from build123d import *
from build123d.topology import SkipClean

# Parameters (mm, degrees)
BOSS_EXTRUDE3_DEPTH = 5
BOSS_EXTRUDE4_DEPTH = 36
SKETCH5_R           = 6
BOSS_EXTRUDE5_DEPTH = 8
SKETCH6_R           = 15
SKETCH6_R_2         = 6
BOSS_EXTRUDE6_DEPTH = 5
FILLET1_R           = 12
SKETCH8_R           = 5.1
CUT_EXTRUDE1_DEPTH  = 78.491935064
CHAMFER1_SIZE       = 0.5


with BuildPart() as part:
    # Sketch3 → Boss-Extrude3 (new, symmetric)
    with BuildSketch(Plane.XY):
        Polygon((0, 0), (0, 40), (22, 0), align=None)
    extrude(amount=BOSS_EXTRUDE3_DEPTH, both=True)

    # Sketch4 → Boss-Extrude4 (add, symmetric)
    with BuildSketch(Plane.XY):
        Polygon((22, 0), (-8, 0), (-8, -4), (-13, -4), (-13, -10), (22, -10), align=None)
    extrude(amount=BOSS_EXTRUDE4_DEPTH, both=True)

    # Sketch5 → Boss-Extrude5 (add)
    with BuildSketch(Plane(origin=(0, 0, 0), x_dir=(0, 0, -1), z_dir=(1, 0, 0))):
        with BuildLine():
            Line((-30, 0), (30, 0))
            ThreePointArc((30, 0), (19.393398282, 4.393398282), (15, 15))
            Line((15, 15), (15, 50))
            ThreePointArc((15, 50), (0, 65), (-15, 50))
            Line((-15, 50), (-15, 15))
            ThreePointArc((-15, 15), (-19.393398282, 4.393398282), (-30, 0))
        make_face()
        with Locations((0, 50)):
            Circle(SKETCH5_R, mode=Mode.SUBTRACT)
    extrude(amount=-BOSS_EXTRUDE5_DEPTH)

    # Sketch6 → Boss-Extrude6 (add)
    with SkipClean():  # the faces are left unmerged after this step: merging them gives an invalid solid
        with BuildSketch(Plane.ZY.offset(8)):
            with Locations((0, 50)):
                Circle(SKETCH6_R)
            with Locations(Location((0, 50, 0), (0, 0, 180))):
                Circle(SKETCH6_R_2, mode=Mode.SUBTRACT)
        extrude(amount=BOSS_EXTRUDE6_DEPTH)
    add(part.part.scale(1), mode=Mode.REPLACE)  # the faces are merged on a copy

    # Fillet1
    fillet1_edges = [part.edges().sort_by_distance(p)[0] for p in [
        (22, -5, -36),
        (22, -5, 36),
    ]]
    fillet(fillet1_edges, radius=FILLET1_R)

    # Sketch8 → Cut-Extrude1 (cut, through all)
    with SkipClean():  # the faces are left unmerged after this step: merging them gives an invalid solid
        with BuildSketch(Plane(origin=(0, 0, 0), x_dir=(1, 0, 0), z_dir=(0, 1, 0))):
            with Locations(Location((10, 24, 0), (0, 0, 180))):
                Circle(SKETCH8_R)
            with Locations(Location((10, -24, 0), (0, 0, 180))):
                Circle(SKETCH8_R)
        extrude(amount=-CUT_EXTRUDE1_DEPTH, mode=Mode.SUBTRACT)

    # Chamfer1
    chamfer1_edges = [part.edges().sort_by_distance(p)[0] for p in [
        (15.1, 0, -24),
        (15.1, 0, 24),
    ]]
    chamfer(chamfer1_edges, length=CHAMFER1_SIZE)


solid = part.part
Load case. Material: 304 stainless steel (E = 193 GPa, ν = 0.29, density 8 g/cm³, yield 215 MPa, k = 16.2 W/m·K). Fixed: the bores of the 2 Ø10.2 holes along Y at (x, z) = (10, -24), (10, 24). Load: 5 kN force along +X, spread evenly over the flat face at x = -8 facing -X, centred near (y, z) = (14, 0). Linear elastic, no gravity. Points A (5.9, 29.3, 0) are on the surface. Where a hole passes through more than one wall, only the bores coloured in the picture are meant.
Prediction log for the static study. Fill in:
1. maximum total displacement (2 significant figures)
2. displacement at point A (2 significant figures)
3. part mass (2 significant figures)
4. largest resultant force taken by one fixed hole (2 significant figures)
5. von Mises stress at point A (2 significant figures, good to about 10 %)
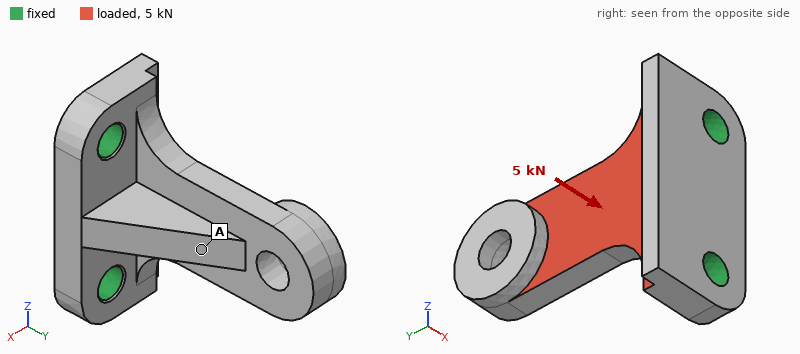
82 µm
38 µm
350 g
2.5 kN
18 MPa
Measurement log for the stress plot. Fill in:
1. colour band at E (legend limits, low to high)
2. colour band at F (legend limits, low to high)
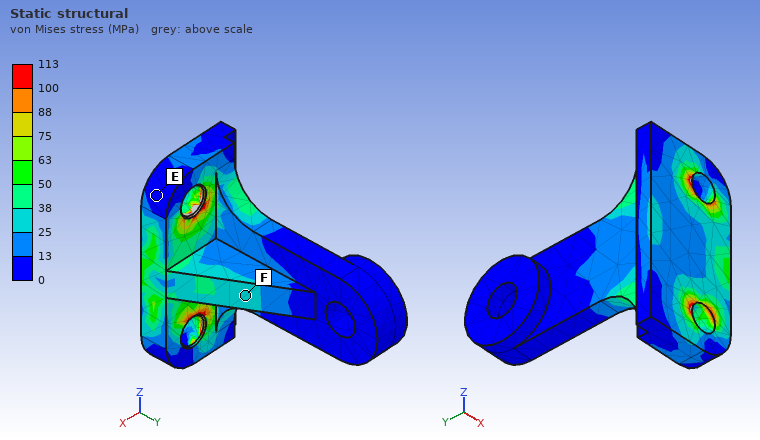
0 to 13 MPa
25 to 38 MPa
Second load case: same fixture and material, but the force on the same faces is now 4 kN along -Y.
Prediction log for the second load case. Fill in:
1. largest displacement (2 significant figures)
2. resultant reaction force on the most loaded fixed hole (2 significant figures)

42 µm
2.0 kN
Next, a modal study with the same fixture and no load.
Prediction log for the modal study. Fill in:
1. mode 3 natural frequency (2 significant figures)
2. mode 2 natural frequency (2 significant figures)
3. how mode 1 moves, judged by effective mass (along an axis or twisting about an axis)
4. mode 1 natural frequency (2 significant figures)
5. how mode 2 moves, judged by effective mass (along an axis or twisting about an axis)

7500 Hz
4200 Hz
along X
2400 Hz
along Z
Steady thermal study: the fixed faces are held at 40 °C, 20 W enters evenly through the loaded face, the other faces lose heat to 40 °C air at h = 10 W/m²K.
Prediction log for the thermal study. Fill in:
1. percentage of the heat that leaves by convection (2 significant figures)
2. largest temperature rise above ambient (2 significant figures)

17 %
64 K
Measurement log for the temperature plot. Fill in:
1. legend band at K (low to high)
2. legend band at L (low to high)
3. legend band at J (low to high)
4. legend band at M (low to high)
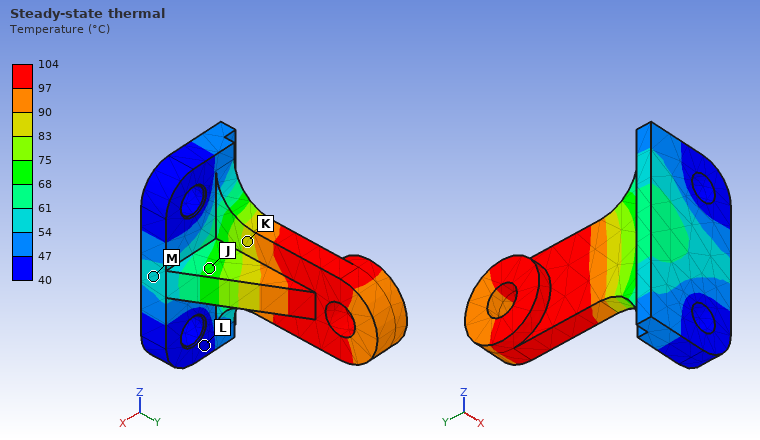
83 to 90 °C
40 to 47 °C
68 to 75 °C
54 to 61 °C
